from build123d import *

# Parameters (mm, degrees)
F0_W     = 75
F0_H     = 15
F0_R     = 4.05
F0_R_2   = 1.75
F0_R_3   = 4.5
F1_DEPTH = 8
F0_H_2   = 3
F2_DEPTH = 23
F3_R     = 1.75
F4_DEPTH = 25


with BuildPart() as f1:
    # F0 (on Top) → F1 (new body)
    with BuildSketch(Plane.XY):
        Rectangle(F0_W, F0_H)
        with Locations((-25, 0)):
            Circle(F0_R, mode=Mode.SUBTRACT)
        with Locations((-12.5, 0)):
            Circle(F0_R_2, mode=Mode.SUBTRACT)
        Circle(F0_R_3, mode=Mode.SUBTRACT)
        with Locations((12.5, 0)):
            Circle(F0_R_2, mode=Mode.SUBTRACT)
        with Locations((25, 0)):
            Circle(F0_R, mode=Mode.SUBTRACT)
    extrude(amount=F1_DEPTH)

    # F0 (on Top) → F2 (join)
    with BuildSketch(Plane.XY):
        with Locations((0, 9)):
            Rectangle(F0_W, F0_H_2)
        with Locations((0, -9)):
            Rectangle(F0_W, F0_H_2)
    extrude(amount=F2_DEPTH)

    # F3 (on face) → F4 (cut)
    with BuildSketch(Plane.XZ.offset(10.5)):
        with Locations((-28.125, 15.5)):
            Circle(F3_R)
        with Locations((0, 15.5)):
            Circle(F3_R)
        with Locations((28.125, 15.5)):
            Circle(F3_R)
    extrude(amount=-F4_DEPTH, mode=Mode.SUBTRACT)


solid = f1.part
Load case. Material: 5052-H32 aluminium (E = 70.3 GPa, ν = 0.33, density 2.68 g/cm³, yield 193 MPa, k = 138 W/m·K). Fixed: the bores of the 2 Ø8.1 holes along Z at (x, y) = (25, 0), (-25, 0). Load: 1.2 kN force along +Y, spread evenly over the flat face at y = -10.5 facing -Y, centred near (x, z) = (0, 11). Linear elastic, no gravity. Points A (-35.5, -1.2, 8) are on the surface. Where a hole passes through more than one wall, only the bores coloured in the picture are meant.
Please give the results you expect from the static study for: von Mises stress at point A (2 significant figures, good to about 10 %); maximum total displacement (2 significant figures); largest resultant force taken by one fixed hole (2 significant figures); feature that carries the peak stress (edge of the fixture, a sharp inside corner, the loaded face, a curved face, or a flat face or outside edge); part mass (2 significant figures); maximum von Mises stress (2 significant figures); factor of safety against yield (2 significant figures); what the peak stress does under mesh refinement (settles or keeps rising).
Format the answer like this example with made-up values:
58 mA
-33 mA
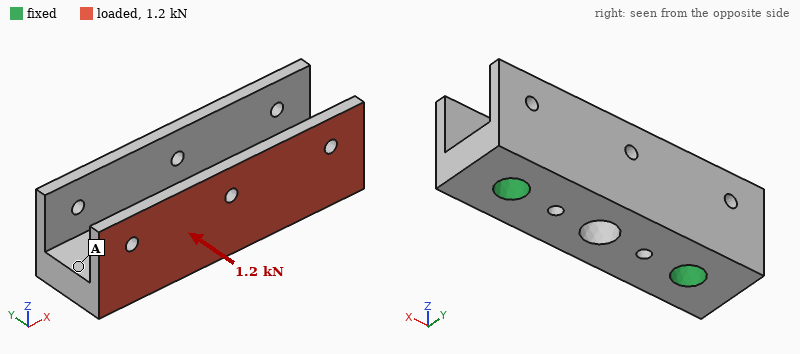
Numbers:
5.3 MPa
50 µm
600 N
the loaded face
47 g
46 MPa
4.2
settles
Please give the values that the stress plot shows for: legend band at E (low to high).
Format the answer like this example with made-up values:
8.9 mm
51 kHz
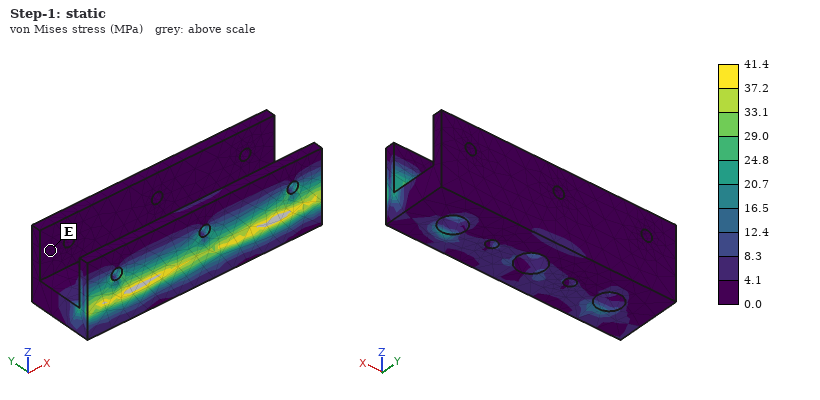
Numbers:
0.0 to 4.1 MPa
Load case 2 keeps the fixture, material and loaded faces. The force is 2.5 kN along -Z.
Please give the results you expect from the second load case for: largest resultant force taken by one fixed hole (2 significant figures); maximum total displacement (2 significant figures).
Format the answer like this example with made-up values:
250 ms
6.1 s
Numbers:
1.3 kN
41 µm
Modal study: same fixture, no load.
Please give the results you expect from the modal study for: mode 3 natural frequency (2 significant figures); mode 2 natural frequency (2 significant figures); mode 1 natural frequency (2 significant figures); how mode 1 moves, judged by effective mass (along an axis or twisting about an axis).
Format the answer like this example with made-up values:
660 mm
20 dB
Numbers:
9700 Hz
8700 Hz
8200 Hz
along Y
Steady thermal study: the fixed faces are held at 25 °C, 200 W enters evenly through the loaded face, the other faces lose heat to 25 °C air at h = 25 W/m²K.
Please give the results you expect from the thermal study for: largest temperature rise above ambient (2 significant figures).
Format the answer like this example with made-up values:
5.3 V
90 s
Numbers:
76 K
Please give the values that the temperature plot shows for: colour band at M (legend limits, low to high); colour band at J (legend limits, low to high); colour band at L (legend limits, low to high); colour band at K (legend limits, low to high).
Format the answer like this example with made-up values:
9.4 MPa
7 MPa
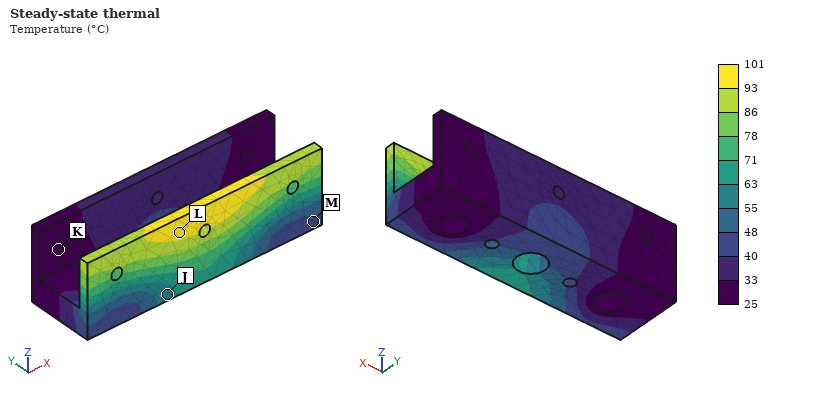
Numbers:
40 to 48 °C
55 to 63 °C
93 to 101 °C
25 to 33 °C
